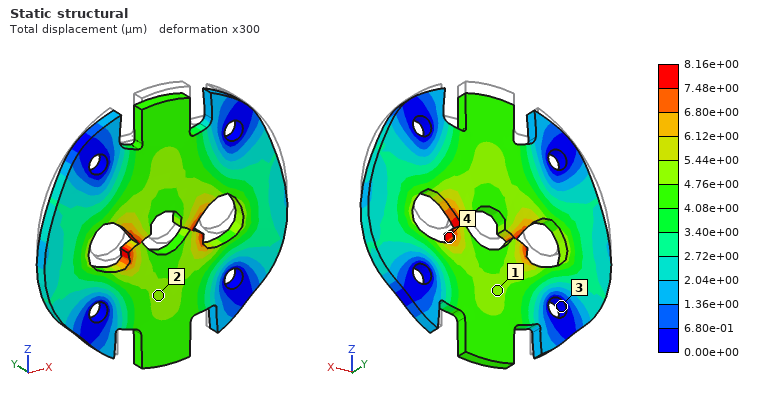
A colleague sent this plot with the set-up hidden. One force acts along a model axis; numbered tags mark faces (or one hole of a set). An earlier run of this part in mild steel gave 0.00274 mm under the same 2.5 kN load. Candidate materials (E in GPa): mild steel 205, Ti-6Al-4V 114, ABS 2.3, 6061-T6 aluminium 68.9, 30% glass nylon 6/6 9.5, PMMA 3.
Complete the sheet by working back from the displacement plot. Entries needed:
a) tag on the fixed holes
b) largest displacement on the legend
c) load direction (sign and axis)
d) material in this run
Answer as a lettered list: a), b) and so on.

a) 3
b) 8.16e+00 µm
c) -Z
d) 6061-T6 aluminium
